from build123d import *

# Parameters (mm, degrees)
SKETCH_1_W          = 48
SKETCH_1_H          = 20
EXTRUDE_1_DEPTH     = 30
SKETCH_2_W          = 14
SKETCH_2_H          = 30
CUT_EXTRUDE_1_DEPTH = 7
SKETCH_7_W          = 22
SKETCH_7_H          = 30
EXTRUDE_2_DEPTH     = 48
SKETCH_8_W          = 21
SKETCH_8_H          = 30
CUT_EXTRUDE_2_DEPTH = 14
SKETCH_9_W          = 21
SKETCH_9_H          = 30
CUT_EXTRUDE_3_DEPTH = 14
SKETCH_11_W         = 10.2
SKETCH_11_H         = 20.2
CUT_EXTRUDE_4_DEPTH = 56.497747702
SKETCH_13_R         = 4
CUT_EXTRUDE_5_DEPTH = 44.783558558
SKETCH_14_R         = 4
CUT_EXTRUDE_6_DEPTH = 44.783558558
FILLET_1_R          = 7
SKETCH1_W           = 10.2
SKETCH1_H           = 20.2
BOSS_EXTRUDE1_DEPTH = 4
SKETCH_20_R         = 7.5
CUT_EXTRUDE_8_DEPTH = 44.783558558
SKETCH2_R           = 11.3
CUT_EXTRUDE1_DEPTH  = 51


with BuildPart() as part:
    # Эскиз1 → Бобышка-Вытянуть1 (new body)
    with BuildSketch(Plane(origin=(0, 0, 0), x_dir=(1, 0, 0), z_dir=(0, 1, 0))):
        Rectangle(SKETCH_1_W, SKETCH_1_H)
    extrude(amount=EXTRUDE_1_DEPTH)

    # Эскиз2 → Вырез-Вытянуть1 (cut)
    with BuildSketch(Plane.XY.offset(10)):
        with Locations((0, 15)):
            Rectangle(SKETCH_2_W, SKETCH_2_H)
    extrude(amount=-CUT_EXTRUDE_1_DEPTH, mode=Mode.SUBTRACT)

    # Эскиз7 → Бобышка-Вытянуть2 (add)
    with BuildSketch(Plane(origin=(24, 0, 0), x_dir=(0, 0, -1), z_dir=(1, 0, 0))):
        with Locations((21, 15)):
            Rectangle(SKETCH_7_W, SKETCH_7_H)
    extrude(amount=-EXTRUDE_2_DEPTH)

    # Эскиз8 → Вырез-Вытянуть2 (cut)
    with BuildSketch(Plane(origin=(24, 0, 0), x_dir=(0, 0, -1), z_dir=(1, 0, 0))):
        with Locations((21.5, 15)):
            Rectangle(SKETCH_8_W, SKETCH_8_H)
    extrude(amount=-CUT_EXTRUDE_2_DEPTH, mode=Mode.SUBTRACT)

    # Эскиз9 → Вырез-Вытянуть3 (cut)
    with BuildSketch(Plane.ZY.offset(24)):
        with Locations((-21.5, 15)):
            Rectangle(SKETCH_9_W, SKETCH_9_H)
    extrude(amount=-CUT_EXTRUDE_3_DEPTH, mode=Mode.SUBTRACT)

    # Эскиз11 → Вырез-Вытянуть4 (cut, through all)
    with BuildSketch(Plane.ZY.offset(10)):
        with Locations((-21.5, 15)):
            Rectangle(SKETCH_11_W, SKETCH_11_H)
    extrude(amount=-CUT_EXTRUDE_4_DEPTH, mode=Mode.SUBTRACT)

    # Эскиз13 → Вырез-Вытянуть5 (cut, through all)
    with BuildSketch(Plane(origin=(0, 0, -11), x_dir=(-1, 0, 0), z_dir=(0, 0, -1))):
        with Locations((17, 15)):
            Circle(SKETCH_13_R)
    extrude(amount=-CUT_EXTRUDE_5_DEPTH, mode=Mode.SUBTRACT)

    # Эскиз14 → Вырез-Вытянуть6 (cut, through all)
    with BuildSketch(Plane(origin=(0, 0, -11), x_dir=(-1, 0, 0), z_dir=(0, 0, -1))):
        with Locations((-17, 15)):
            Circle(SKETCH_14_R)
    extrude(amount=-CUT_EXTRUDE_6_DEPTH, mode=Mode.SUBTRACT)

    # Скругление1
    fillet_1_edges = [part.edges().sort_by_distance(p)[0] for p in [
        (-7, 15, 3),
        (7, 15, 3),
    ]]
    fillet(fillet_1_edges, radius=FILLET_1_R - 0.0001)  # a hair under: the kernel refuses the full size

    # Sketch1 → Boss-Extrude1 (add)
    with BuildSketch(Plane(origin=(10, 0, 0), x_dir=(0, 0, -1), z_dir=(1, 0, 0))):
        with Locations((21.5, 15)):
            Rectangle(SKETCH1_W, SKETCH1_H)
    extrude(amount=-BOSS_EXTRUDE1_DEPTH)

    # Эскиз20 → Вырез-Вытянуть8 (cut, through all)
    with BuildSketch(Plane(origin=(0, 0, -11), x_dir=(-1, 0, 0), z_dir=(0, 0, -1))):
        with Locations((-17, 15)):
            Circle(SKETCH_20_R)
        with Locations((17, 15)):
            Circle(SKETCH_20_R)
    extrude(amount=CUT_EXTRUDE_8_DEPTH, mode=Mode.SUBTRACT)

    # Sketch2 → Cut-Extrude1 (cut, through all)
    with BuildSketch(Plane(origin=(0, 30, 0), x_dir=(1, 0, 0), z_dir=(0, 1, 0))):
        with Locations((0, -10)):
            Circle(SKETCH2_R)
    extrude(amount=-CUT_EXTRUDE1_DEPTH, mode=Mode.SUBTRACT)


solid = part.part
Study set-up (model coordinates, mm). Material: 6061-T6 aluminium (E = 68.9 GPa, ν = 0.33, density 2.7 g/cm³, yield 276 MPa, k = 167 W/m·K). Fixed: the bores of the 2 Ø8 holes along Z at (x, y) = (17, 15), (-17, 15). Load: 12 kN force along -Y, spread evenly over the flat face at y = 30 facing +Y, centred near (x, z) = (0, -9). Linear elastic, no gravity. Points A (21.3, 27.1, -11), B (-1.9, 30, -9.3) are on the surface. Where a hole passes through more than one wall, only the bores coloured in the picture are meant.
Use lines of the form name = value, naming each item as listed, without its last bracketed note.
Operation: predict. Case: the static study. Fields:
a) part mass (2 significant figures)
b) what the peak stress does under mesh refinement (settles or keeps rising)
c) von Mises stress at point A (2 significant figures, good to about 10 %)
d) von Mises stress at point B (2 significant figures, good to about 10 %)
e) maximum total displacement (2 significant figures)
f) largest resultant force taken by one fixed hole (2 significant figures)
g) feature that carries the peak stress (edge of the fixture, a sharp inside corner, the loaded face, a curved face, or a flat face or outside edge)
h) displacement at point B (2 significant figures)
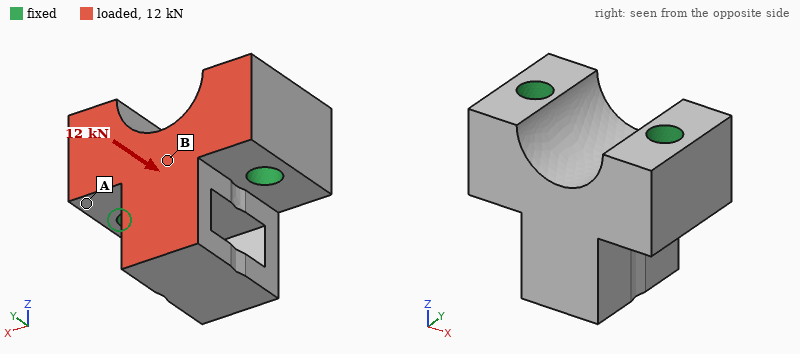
part mass = 85 g
what the peak stress does under mesh refinement = keeps rising
von Mises stress at point A = 9.6 MPa
von Mises stress at point B = 27 MPa
maximum total displacement = 48 µm
largest resultant force taken by one fixed hole = 6.0 kN
feature that carries the peak stress = edge of the fixture
displacement at point B = 14 µm
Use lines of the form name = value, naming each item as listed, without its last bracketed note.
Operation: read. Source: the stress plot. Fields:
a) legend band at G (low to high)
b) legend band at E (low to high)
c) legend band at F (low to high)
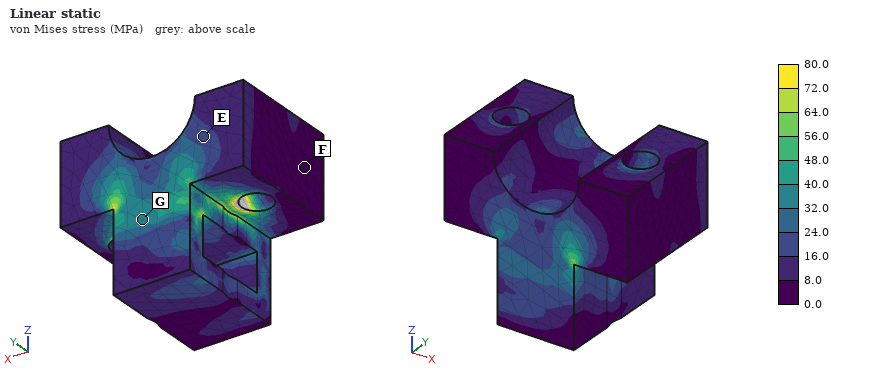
legend band at G = 32.0 to 40.0 MPa
legend band at E = 16.0 to 24.0 MPa
legend band at F = 0.0 to 8.0 MPa
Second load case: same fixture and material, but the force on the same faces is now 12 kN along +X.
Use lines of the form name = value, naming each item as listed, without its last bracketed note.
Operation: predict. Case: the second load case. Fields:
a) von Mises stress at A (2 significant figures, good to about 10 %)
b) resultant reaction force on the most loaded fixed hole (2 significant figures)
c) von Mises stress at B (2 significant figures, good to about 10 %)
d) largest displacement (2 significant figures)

von Mises stress at A = 10 MPa
resultant reaction force on the most loaded fixed hole = 7.6 kN
von Mises stress at B = 29 MPa
largest displacement = 53 µm
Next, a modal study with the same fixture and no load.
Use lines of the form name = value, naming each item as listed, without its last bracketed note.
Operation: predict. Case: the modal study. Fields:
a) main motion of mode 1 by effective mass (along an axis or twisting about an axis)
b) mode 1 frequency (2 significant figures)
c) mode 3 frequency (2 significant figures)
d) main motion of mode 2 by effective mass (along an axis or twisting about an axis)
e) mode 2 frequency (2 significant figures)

main motion of mode 1 by effective mass = along Y
mode 1 frequency = 12 kHz
mode 3 frequency = 22 kHz
main motion of mode 2 by effective mass = along X
mode 2 frequency = 15 kHz
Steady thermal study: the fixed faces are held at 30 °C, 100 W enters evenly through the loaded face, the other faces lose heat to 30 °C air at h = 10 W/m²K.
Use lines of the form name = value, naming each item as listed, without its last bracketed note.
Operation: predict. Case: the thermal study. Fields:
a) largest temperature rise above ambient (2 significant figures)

largest temperature rise above ambient = 20 K
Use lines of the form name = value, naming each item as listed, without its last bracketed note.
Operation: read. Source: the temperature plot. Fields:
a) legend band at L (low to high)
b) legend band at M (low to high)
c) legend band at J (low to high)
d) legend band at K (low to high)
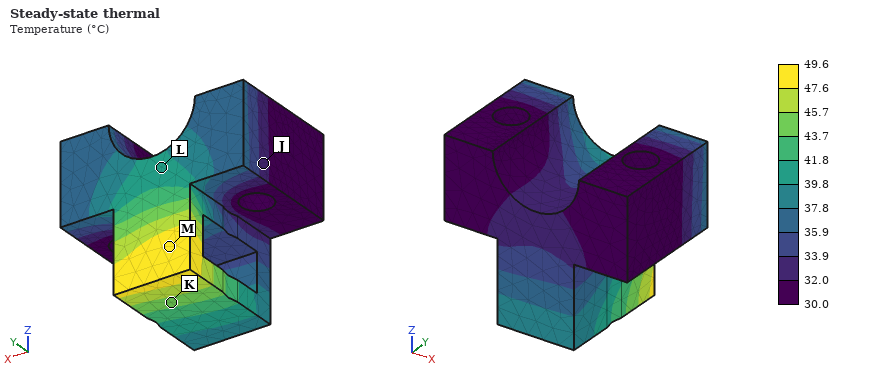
legend band at L = 39.8 to 41.8 °C
legend band at M = 47.6 to 49.6 °C
legend band at J = 32.0 to 33.9 °C
legend band at K = 43.7 to 45.7 °C
